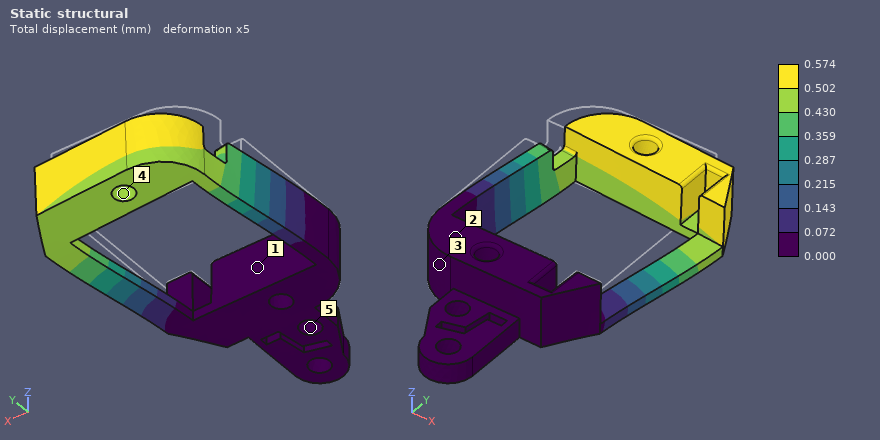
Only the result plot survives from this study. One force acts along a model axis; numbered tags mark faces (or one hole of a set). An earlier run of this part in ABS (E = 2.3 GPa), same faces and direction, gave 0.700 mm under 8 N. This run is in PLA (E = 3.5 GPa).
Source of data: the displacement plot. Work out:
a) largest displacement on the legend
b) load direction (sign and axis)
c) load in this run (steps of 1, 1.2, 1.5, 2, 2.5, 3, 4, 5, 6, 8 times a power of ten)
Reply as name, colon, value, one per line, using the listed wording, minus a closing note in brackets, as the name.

largest displacement on the legend: 0.574 mm
load direction: +X
load in this run: 10 N
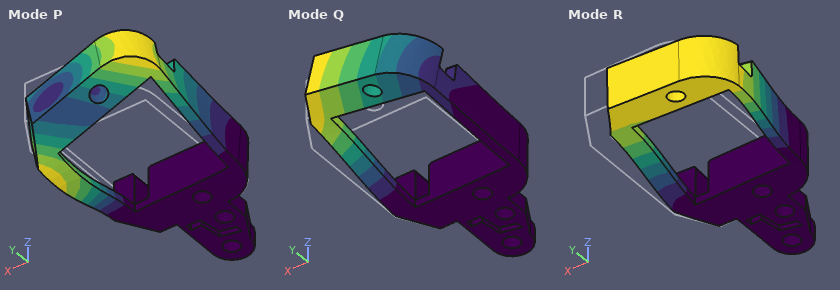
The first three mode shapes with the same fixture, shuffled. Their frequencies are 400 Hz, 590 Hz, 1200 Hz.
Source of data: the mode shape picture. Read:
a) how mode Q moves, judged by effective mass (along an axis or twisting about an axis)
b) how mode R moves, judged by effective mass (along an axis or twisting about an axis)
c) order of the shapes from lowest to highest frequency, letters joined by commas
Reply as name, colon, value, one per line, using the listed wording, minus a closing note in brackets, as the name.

how mode Q moves, judged by effective mass: along Z
how mode R moves, judged by effective mass: along X
order of the shapes from lowest to highest frequency, letters joined by commas: Q, R, P
